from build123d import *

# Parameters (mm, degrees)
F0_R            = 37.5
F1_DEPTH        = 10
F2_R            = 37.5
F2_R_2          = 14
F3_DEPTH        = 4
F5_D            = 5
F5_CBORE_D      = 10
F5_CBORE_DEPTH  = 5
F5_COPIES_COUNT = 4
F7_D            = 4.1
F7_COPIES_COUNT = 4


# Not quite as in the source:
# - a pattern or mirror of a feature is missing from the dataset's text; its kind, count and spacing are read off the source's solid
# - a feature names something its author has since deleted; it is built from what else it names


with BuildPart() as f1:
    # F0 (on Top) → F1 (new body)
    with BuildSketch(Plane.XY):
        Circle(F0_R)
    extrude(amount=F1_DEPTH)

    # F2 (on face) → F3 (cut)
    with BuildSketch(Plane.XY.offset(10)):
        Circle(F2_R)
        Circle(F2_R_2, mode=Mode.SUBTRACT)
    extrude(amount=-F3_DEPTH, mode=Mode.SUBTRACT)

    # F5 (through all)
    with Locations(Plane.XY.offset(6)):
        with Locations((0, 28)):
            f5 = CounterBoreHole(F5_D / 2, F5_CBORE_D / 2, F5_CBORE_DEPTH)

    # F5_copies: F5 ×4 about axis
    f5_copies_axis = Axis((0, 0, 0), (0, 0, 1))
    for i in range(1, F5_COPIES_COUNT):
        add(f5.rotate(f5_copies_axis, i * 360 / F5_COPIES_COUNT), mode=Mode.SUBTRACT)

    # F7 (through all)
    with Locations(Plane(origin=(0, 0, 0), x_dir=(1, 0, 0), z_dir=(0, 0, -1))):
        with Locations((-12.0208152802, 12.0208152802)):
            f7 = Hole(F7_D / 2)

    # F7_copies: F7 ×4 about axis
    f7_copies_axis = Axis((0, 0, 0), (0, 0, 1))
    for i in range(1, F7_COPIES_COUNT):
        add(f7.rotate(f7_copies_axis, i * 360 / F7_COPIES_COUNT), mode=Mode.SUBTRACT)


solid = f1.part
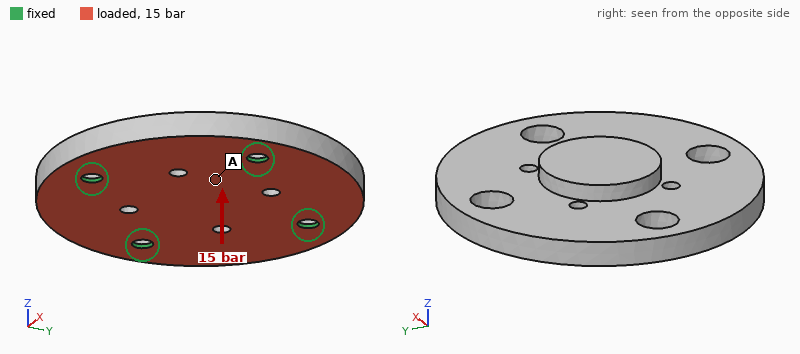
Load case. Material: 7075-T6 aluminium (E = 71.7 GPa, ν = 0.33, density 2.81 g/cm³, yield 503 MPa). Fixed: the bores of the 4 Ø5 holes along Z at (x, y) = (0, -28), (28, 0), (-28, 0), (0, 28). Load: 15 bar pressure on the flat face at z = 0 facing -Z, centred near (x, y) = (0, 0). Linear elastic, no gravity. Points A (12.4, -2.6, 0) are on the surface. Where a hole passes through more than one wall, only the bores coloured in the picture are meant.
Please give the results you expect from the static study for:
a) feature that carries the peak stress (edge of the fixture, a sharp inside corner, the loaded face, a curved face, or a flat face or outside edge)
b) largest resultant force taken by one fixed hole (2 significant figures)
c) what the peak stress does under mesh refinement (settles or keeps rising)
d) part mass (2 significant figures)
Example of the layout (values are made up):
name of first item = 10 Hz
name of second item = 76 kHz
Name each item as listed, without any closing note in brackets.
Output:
feature that carries the peak stress = edge of the fixture
largest resultant force taken by one fixed hole = 1.7 kN
what the peak stress does under mesh refinement = keeps rising
part mass = 76 g
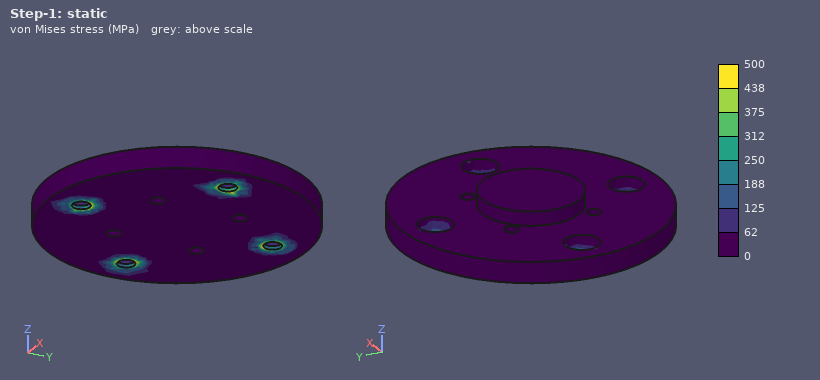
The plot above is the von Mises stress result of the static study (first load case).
